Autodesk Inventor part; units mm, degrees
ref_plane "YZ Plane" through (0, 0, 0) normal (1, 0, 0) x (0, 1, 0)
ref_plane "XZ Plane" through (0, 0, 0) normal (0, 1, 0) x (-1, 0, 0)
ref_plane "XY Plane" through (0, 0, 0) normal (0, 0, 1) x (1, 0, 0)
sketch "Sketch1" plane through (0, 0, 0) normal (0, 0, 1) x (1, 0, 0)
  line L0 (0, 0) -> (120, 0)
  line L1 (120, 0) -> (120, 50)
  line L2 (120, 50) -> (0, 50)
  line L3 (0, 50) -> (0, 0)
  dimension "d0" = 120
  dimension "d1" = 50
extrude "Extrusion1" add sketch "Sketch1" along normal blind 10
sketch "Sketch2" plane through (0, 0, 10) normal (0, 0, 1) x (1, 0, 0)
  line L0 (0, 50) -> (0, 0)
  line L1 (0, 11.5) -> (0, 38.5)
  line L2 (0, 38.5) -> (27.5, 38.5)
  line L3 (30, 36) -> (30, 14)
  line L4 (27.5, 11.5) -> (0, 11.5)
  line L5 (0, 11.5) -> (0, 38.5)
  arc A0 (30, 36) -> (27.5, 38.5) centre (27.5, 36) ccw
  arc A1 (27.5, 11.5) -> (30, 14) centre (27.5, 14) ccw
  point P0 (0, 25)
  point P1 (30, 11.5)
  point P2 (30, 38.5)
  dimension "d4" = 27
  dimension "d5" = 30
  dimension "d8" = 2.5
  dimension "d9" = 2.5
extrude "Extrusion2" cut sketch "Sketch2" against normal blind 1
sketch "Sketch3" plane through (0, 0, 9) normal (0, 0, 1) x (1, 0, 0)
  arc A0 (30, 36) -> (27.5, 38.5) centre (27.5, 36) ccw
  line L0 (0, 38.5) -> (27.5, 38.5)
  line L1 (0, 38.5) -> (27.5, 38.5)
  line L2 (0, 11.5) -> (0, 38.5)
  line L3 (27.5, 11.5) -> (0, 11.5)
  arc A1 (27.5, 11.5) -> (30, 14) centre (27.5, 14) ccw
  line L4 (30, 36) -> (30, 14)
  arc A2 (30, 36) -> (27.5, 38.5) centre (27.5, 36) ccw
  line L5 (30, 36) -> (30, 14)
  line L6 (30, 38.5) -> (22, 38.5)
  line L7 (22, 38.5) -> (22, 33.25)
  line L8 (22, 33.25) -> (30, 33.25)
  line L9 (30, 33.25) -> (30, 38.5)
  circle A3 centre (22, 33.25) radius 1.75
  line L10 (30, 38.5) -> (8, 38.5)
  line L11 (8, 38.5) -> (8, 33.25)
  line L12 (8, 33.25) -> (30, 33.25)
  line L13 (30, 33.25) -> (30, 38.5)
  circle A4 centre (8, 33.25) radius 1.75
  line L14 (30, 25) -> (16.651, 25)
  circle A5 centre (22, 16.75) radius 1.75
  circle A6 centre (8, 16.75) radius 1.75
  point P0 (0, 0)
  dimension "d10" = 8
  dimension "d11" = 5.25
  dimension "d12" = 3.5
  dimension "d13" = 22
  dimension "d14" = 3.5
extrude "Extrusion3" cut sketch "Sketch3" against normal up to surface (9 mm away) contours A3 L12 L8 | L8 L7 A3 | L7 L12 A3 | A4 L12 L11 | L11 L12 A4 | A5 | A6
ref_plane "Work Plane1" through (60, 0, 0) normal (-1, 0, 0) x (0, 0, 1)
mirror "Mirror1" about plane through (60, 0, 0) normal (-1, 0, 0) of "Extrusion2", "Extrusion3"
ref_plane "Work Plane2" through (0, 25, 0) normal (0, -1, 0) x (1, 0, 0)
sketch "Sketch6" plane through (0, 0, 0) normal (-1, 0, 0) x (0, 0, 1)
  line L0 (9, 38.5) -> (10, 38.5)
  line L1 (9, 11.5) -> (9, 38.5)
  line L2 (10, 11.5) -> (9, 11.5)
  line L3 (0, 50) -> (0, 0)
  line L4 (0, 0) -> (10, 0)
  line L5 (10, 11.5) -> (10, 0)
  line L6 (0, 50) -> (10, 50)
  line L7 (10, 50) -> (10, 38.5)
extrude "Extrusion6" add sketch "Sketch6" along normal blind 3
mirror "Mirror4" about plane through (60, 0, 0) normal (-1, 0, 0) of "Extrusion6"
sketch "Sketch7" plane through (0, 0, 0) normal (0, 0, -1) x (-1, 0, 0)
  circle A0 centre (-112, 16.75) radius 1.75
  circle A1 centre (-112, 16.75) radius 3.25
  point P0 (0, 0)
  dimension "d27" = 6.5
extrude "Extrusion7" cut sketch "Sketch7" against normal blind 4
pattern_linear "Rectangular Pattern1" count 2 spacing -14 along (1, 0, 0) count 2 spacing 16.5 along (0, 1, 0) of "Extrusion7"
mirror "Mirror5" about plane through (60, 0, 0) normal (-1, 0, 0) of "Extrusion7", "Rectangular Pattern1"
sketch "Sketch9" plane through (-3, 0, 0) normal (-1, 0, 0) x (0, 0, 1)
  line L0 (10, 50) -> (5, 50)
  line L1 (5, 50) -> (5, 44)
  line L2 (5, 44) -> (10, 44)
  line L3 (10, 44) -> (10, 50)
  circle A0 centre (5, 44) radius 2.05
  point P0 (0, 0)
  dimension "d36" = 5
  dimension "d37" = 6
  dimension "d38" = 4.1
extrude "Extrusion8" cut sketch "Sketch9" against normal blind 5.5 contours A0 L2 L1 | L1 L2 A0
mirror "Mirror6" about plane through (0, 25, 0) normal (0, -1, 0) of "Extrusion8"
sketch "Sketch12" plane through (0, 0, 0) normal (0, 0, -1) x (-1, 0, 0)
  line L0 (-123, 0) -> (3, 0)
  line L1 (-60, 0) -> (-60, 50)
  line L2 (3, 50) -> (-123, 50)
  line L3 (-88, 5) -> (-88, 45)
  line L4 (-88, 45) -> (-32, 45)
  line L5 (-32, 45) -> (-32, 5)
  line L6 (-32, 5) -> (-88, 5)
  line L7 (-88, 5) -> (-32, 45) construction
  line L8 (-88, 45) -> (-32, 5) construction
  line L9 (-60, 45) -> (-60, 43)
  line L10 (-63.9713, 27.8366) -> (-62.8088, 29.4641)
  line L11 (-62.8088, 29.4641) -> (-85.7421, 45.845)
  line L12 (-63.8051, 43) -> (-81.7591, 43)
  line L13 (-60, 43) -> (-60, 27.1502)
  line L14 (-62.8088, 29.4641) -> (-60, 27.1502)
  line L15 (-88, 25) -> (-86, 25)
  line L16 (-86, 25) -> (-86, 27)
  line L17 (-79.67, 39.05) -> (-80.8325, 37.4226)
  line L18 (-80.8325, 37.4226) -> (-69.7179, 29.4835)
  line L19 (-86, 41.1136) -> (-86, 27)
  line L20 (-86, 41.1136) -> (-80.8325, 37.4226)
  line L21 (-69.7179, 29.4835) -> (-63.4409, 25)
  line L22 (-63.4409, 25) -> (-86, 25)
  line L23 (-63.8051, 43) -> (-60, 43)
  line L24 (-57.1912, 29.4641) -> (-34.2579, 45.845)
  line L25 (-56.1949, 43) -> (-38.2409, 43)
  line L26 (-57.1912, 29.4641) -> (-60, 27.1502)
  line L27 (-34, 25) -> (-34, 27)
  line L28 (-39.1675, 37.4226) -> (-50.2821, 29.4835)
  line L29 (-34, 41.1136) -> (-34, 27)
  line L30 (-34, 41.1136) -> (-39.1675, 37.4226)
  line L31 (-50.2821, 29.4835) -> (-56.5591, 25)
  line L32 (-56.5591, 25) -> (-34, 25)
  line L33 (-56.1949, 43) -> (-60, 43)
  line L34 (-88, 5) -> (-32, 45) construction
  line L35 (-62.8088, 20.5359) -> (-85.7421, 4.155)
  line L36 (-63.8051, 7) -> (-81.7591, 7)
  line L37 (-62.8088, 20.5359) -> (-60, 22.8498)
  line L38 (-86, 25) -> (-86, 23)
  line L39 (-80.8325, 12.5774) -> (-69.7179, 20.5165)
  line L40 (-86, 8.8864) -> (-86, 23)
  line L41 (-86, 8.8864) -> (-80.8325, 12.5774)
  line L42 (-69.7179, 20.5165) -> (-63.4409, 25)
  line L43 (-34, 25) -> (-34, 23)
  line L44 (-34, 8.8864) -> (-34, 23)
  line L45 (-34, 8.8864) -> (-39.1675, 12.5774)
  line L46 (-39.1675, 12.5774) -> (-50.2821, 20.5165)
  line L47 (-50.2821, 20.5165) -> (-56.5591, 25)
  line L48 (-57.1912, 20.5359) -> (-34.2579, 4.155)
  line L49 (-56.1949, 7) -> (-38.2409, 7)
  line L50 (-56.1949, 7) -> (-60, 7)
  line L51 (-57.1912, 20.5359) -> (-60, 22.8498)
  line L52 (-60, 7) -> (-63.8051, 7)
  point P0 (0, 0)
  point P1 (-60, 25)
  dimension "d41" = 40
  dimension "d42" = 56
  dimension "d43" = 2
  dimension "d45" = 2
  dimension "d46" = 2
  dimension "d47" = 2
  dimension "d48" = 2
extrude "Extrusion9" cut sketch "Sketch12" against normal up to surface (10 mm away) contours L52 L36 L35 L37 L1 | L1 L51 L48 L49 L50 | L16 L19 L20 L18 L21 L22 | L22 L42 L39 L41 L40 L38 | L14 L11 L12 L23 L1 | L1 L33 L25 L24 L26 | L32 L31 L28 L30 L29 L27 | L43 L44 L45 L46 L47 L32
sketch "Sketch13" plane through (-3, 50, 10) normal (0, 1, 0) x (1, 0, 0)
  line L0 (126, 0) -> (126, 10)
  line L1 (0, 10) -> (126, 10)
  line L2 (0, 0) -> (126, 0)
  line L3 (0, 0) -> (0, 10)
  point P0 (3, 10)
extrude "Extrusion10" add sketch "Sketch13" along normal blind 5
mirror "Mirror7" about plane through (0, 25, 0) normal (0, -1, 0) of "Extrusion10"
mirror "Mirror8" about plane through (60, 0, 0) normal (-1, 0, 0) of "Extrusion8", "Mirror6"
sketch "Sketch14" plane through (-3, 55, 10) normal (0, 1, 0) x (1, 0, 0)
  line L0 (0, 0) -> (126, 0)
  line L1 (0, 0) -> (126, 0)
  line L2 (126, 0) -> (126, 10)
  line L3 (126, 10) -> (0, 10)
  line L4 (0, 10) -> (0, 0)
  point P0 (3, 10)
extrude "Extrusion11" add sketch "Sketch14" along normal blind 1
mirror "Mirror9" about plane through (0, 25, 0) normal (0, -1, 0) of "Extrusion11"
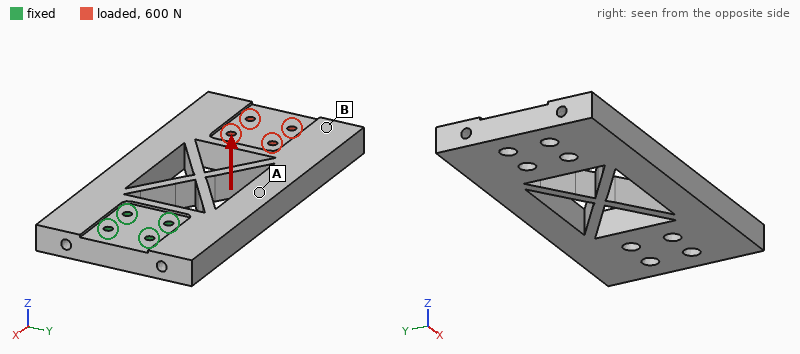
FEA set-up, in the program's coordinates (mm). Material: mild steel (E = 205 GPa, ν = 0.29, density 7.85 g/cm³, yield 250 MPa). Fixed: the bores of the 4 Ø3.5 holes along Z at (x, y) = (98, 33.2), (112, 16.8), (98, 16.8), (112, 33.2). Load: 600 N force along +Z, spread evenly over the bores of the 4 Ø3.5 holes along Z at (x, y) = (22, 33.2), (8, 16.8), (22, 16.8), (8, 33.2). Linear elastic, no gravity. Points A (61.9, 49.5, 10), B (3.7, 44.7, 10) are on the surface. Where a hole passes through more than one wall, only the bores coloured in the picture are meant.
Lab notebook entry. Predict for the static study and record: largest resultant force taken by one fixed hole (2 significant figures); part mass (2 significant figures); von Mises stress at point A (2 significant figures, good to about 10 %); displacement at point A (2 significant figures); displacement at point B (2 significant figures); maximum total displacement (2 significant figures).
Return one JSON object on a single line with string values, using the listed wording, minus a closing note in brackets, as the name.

{"largest resultant force taken by one fixed hole": "1.6 kN", "part mass": "480 g", "von Mises stress at point A": "54 MPa", "displacement at point A": "0.070 mm", "displacement at point B": "0.30 mm", "maximum total displacement": "0.33 mm"}
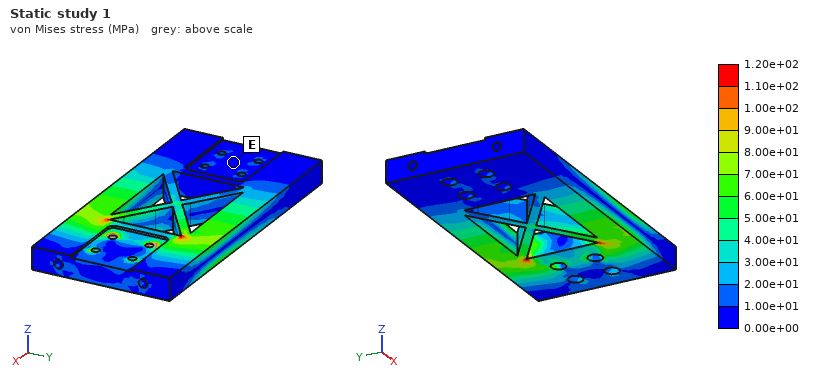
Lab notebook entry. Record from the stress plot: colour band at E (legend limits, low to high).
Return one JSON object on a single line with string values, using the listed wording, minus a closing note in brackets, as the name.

{"colour band at E": "0.00e+00 to 1.00e+01 MPa"}
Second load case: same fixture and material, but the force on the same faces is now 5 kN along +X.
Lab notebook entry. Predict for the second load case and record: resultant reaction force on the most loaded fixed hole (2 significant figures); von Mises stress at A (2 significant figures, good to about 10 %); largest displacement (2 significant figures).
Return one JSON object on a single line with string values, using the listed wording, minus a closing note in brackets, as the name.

{"resultant reaction force on the most loaded fixed hole": "1.5 kN", "von Mises stress at A": "32 MPa", "largest displacement": "73 µm"}
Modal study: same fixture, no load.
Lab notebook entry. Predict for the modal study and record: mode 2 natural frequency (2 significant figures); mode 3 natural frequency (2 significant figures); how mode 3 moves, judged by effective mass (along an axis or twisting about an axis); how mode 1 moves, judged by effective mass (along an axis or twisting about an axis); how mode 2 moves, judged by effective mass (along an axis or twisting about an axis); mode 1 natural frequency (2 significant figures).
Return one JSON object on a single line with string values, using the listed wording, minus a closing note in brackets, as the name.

{"mode 2 natural frequency": "1800 Hz", "mode 3 natural frequency": "2200 Hz", "how mode 3 moves, judged by effective mass": "along Y", "how mode 1 moves, judged by effective mass": "along Z", "how mode 2 moves, judged by effective mass": "twisting about X", "mode 1 natural frequency": "570 Hz"}
